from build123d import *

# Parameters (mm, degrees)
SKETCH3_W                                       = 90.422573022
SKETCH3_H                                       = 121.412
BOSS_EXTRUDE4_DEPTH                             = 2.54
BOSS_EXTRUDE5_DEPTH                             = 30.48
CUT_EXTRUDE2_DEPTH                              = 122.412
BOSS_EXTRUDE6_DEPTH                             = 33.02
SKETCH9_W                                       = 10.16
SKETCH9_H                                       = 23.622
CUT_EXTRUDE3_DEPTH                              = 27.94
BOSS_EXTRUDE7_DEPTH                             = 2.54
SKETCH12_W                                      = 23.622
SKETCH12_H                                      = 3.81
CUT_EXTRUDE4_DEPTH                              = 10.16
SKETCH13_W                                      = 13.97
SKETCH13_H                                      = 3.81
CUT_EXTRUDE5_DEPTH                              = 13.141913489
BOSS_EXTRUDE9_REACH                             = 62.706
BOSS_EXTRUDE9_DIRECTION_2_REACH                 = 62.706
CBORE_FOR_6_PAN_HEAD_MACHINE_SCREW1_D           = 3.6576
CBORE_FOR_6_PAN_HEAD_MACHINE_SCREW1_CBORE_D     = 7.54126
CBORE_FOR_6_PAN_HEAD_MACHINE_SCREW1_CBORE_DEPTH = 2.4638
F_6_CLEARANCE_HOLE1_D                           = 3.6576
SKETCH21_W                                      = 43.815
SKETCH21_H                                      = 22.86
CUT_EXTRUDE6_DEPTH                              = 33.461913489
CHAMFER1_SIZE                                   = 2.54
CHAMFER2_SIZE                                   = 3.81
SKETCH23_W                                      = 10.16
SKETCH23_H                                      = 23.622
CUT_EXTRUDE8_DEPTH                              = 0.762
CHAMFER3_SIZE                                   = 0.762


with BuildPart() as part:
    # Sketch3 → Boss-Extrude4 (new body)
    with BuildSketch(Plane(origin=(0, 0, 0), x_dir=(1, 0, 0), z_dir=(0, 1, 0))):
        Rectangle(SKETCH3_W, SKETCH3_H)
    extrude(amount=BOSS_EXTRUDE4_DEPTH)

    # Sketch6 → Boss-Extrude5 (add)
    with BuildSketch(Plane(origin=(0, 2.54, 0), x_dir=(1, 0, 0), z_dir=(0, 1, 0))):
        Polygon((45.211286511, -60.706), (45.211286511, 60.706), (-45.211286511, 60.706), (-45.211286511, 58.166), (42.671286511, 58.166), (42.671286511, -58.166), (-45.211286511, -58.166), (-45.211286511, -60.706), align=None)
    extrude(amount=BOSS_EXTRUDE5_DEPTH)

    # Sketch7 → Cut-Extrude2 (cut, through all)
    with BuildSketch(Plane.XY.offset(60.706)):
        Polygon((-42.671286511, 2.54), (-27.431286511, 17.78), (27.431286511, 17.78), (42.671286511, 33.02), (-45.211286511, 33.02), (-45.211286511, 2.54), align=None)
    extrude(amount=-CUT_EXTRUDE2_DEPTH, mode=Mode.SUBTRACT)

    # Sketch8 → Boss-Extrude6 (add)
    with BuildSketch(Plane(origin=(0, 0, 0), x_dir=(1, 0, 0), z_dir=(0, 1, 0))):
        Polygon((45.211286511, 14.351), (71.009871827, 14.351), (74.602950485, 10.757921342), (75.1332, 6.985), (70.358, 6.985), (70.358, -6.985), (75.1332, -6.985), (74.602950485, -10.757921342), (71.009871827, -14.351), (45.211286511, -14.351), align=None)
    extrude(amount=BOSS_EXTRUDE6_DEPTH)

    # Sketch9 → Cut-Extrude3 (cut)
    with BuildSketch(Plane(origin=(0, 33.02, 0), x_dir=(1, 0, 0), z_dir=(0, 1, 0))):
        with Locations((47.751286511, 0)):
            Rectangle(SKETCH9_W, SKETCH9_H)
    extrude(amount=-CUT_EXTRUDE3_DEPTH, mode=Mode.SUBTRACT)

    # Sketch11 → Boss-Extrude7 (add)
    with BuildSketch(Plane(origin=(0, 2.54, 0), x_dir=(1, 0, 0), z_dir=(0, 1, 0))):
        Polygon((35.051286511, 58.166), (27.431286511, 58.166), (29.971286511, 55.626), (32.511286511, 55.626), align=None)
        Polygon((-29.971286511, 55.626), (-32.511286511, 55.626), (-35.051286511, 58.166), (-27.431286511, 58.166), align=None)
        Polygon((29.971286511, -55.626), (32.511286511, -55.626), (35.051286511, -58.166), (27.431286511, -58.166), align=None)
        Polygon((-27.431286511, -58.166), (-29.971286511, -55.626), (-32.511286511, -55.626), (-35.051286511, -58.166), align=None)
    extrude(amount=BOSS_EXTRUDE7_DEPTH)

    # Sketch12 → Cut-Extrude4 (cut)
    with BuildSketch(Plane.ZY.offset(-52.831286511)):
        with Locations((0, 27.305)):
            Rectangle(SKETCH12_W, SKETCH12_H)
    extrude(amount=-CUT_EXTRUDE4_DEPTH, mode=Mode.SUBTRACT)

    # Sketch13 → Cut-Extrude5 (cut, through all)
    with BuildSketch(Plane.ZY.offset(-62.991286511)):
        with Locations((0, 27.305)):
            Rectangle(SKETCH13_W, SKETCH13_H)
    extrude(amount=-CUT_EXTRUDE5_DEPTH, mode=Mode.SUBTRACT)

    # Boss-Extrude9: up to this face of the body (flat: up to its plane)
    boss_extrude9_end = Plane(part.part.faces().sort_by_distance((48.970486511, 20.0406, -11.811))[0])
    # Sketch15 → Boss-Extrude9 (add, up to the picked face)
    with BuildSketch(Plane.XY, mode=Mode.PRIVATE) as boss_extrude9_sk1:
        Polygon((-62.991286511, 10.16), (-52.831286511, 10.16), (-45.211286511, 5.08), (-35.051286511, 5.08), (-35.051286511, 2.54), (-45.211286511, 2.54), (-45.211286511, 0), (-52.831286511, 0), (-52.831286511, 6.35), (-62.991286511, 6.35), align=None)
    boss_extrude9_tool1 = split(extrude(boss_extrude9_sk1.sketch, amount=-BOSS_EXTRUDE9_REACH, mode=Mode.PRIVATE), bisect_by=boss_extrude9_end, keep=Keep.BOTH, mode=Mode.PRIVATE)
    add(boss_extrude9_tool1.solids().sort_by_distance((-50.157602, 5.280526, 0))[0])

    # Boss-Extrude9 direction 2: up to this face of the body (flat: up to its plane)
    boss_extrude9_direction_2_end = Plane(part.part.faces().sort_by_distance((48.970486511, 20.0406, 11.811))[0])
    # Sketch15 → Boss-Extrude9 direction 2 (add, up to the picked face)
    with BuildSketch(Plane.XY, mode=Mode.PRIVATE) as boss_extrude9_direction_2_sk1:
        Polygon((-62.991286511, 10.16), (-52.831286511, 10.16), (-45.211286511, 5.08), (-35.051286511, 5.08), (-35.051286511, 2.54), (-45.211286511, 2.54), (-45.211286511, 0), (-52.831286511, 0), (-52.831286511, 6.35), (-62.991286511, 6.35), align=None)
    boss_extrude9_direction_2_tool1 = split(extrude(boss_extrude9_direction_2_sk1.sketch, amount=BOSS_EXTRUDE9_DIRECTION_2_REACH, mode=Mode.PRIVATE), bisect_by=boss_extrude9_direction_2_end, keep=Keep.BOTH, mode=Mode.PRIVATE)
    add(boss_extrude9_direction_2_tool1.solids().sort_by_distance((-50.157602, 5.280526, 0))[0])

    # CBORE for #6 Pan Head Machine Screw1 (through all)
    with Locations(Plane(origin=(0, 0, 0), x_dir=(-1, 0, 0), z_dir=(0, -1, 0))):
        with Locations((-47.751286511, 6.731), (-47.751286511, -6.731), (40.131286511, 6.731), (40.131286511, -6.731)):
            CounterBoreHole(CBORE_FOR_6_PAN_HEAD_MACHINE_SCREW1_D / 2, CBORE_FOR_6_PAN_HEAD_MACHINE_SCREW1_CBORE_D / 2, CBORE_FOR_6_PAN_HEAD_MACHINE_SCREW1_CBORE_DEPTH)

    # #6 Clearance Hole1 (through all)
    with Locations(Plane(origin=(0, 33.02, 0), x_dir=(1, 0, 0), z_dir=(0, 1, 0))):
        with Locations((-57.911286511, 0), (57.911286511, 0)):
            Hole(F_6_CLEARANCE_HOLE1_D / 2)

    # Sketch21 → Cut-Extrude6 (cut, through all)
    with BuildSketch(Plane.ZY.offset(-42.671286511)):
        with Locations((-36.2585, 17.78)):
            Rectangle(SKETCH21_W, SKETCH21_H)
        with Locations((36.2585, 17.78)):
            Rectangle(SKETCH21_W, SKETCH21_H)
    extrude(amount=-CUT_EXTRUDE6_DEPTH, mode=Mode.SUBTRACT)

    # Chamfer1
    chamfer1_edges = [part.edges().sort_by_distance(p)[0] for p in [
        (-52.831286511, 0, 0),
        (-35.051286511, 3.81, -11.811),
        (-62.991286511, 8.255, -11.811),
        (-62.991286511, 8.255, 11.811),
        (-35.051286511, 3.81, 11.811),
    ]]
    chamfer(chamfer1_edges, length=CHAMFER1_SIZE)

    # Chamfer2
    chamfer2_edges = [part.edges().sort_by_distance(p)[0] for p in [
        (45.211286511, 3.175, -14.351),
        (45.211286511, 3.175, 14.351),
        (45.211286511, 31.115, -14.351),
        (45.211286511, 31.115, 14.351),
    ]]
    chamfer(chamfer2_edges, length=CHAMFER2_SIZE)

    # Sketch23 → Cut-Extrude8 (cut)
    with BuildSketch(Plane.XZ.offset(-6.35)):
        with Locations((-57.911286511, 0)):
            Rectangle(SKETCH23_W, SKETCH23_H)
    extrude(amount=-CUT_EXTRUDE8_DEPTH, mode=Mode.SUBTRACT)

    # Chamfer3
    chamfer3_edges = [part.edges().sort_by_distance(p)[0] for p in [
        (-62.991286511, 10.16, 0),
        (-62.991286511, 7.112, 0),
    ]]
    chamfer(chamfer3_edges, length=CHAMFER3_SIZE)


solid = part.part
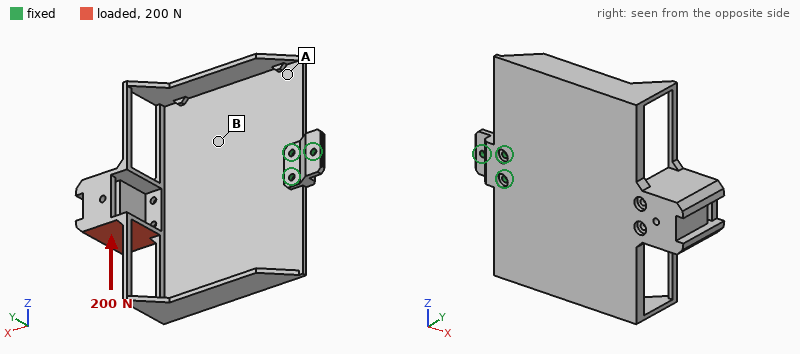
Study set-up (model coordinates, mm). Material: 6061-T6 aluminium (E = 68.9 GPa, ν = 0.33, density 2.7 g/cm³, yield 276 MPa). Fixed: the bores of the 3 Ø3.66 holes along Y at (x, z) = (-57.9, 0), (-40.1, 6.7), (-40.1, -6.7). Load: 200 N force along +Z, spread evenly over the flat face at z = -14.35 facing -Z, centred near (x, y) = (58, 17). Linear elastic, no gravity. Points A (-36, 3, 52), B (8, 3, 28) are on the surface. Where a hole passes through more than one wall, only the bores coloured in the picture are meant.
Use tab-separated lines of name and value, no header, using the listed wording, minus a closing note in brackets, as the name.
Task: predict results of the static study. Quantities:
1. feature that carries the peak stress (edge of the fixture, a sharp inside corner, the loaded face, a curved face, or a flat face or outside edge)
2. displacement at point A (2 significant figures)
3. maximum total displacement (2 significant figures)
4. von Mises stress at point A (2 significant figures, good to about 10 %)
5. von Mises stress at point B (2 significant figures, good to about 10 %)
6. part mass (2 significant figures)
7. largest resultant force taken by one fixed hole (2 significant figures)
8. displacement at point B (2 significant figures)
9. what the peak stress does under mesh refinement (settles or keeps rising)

feature that carries the peak stress	edge of the fixture
displacement at point A	0.32 mm
maximum total displacement	1.1 mm
von Mises stress at point A	6.0 MPa
von Mises stress at point B	13 MPa
part mass	160 g
largest resultant force taken by one fixed hole	810 N
displacement at point B	0.30 mm
what the peak stress does under mesh refinement	keeps rising
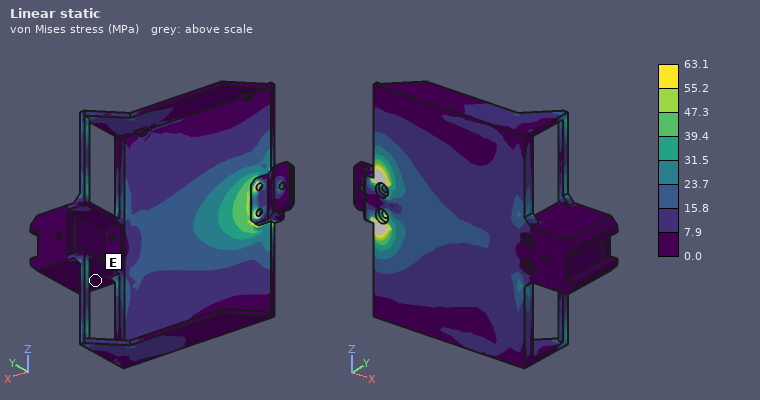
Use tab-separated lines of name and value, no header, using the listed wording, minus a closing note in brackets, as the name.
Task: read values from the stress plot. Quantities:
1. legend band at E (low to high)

legend band at E	0.0 to 7.9 MPa
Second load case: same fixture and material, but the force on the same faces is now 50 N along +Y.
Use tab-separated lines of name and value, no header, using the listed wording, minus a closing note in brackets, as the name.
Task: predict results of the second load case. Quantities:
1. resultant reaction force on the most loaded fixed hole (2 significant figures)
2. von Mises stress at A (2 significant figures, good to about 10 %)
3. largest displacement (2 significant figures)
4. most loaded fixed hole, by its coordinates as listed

resultant reaction force on the most loaded fixed hole	250 N
von Mises stress at A	19 MPa
largest displacement	2.0 mm
most loaded fixed hole, by its coordinates as listed	(-57.9, 0)
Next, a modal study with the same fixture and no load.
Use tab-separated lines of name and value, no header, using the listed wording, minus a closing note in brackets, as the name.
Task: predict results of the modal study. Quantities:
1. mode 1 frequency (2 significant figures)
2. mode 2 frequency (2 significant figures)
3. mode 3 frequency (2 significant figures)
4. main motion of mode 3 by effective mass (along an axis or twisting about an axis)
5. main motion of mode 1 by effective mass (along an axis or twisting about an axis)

mode 1 frequency	100 Hz
mode 2 frequency	210 Hz
mode 3 frequency	550 Hz
main motion of mode 3 by effective mass	along Y
main motion of mode 1 by effective mass	along Y
